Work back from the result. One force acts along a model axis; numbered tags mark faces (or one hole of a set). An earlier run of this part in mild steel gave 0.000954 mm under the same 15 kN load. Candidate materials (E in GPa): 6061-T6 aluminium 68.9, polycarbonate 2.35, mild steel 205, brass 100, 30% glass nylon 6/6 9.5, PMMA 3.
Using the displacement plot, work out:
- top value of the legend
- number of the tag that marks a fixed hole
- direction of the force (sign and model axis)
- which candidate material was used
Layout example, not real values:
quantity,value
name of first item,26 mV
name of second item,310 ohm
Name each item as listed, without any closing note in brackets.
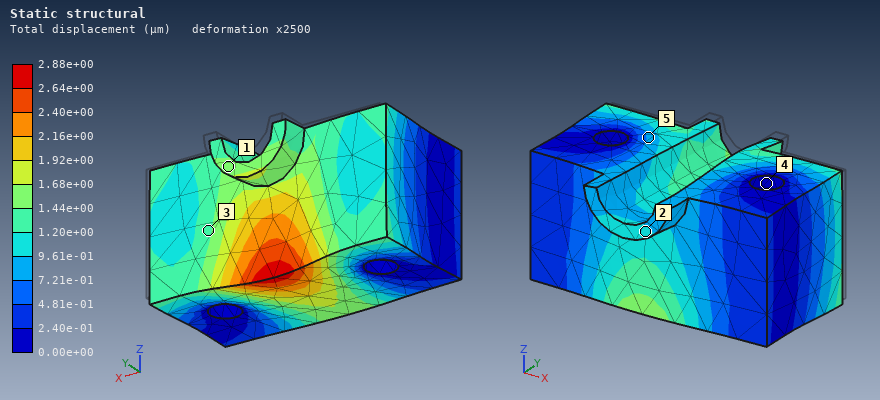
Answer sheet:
quantity,value
top value of the legend,2.88e+00 µm
number of the tag that marks a fixed hole,4
direction of the force,-Y
which candidate material was used,6061-T6 aluminium
